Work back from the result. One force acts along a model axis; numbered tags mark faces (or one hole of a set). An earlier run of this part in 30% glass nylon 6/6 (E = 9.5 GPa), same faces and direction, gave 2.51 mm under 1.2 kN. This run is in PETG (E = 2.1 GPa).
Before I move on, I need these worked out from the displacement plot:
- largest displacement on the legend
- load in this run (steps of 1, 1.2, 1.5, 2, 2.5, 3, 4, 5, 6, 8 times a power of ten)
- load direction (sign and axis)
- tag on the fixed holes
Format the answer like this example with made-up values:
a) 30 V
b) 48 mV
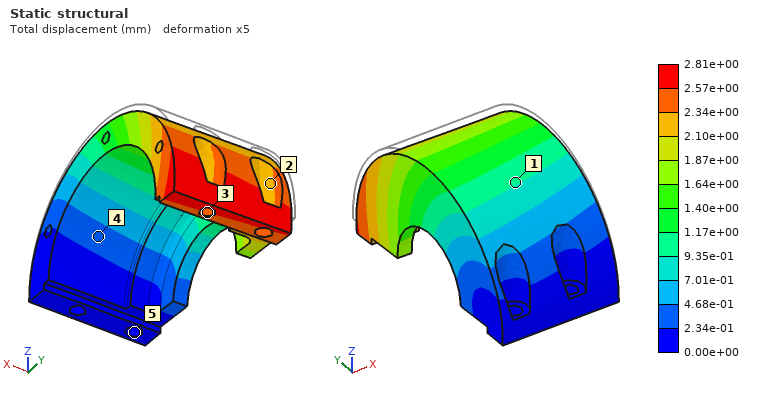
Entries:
a) 2.81e+00 mm
b) 300 N
c) -Z
d) 5
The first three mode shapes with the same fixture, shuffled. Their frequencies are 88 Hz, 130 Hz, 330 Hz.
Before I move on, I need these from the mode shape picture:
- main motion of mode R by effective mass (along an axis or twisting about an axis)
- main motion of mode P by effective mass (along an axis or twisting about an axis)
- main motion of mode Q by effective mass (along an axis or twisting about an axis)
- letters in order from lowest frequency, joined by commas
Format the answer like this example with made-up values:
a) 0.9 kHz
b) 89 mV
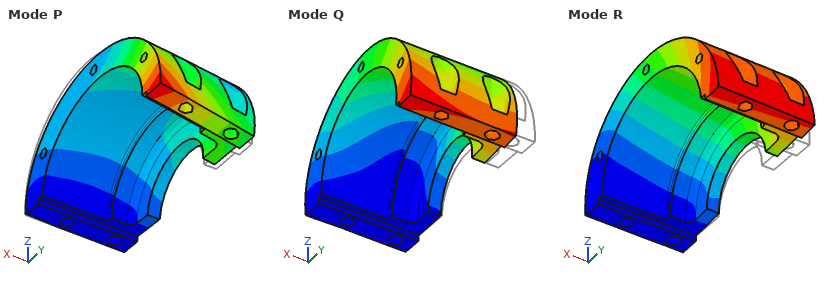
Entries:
a) along Z
b) along Y
c) along X
d) R, Q, P
